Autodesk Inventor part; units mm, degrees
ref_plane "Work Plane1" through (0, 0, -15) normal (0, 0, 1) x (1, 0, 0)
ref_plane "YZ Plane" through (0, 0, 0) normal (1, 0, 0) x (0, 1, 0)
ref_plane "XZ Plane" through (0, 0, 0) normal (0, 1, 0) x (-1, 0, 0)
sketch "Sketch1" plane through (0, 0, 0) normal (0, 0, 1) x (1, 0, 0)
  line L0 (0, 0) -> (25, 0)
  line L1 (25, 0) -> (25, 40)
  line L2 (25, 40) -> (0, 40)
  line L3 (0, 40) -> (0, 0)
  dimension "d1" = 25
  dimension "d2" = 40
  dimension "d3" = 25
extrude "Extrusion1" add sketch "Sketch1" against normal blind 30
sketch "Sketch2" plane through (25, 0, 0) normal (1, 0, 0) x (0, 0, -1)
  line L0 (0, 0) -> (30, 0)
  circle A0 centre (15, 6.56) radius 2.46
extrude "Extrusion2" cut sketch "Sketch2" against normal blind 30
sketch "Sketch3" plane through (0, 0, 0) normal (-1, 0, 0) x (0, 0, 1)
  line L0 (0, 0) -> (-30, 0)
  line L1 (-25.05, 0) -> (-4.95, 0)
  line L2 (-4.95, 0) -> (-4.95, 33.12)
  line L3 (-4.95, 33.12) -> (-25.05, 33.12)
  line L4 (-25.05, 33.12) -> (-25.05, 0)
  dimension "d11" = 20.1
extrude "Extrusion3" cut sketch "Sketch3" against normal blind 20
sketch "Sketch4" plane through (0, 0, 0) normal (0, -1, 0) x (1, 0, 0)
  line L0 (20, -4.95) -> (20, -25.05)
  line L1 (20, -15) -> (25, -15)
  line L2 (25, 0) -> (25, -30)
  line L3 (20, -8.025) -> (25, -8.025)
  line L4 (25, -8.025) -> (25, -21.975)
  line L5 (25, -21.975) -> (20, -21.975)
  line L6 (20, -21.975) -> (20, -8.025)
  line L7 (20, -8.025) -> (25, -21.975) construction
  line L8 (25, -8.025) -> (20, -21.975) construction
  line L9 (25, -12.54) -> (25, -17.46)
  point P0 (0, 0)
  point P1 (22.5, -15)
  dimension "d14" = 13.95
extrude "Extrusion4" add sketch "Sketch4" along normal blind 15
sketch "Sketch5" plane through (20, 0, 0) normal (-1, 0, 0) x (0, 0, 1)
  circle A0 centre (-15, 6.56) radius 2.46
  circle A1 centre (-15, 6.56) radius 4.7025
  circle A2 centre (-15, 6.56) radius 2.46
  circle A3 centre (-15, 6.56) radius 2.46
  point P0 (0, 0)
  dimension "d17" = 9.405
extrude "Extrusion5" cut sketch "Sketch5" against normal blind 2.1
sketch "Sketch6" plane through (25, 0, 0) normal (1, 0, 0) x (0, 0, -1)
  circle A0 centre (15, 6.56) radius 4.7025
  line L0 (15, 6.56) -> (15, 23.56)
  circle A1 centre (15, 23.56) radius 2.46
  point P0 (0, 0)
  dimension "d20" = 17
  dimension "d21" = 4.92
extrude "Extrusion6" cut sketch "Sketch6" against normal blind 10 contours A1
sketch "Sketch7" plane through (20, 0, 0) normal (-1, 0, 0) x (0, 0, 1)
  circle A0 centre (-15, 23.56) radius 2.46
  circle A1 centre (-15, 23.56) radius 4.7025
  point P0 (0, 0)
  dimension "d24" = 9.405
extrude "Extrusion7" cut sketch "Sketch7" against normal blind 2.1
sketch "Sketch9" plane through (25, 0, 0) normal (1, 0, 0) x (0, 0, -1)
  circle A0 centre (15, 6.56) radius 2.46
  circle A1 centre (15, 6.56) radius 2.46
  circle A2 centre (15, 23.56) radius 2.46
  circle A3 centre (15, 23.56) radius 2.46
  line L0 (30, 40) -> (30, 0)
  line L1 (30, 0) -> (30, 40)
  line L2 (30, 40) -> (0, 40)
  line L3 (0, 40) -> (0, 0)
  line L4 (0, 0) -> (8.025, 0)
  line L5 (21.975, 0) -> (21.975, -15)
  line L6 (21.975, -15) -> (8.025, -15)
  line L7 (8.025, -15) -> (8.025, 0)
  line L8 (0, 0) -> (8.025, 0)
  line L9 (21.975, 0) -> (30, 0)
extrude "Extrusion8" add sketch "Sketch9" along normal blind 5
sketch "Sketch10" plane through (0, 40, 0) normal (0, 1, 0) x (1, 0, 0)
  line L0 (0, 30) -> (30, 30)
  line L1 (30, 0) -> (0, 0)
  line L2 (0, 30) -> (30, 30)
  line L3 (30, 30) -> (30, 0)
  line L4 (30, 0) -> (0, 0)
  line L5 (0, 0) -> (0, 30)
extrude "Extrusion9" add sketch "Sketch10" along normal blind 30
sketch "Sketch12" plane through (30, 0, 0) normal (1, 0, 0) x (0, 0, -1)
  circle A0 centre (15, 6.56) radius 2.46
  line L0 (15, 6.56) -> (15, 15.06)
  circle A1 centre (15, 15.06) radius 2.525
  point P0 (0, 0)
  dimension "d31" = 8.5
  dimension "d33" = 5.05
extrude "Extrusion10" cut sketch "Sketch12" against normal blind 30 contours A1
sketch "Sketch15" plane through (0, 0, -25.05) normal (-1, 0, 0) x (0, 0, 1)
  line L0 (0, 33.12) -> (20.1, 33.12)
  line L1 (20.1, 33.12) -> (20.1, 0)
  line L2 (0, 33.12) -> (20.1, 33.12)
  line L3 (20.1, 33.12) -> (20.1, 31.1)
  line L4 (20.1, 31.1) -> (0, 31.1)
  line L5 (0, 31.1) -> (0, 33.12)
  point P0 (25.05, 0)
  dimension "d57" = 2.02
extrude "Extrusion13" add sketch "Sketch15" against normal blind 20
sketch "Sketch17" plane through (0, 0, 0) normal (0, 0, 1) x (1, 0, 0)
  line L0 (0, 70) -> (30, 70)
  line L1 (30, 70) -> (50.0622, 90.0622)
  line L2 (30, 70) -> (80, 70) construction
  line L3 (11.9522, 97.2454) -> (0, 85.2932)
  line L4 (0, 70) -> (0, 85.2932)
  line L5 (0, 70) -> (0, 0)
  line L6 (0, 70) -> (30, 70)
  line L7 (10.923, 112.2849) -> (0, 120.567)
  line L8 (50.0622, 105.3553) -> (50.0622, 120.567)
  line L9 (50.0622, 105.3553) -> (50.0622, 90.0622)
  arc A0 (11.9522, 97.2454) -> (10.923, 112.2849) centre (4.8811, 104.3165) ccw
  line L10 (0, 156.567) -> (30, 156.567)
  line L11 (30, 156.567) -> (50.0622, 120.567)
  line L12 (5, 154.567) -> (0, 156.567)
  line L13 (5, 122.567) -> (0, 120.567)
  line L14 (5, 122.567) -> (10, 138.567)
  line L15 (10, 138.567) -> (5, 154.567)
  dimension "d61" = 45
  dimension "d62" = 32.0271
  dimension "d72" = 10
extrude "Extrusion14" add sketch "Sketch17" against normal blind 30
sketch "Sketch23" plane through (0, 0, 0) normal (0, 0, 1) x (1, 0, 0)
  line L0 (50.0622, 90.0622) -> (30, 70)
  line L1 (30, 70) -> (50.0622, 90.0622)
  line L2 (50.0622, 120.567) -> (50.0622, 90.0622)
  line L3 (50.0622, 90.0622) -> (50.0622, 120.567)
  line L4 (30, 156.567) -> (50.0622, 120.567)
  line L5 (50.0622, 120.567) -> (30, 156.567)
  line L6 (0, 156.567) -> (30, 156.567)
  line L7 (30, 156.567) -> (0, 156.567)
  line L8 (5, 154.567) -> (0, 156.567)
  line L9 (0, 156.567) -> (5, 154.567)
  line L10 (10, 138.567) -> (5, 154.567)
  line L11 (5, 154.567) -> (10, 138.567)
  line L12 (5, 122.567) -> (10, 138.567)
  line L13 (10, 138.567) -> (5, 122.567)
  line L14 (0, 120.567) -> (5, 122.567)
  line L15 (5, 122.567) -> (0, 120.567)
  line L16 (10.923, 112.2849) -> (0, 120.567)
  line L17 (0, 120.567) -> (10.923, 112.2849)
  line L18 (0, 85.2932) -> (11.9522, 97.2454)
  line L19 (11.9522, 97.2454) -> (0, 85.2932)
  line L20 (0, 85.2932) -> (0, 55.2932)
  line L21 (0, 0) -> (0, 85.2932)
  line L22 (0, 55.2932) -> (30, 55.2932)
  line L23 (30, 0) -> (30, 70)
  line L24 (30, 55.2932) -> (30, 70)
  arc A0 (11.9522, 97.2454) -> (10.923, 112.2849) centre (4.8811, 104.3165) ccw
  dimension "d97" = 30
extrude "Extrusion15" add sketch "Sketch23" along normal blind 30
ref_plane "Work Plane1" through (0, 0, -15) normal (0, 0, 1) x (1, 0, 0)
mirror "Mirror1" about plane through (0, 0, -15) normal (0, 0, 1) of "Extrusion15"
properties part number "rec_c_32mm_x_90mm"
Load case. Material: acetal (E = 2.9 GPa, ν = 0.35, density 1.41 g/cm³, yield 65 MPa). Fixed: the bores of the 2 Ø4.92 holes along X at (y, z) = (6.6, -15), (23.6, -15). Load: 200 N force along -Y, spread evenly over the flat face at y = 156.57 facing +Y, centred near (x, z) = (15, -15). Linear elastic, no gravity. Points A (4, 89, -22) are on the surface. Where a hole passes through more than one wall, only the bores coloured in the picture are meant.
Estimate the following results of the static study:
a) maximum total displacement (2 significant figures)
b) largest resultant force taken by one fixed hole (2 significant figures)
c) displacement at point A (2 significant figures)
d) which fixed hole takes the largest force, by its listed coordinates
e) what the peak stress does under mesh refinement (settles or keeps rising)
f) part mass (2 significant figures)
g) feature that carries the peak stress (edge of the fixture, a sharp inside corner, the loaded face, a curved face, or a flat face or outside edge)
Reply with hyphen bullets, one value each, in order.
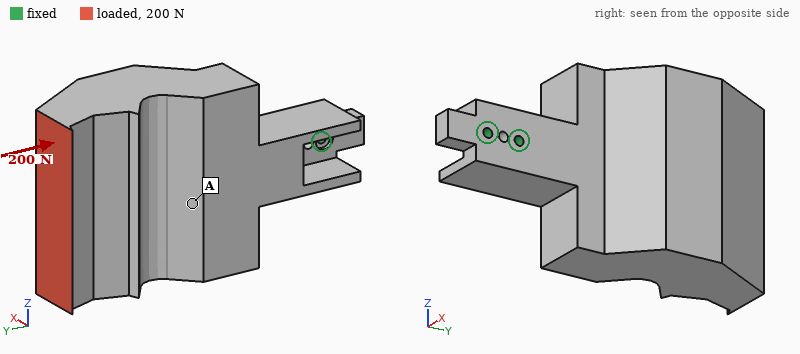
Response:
- 0.16 mm
- 150 N
- 0.077 mm
- (23.6, -15)
- keeps rising
- 520 g
- edge of the fixture
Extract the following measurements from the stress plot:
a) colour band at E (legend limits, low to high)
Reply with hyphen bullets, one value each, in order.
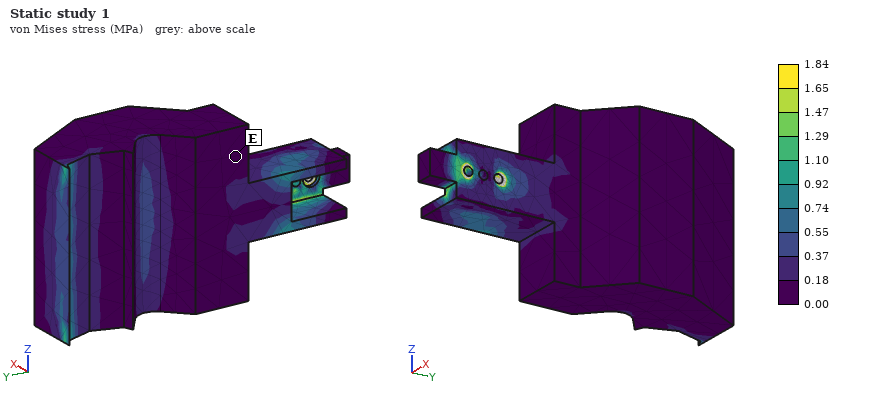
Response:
- 0.00 to 0.18 MPa
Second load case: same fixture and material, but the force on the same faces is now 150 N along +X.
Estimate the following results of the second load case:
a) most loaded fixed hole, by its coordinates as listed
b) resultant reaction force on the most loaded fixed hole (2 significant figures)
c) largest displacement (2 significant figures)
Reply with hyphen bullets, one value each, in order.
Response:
- (23.6, -15)
- 950 N
- 1.8 mm
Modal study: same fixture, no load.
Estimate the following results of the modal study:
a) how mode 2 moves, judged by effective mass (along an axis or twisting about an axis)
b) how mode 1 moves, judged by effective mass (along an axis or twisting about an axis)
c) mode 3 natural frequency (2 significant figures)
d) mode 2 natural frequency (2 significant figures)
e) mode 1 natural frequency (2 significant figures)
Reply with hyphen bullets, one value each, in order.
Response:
- along Z
- along X
- 220 Hz
- 120 Hz
- 110 Hz
